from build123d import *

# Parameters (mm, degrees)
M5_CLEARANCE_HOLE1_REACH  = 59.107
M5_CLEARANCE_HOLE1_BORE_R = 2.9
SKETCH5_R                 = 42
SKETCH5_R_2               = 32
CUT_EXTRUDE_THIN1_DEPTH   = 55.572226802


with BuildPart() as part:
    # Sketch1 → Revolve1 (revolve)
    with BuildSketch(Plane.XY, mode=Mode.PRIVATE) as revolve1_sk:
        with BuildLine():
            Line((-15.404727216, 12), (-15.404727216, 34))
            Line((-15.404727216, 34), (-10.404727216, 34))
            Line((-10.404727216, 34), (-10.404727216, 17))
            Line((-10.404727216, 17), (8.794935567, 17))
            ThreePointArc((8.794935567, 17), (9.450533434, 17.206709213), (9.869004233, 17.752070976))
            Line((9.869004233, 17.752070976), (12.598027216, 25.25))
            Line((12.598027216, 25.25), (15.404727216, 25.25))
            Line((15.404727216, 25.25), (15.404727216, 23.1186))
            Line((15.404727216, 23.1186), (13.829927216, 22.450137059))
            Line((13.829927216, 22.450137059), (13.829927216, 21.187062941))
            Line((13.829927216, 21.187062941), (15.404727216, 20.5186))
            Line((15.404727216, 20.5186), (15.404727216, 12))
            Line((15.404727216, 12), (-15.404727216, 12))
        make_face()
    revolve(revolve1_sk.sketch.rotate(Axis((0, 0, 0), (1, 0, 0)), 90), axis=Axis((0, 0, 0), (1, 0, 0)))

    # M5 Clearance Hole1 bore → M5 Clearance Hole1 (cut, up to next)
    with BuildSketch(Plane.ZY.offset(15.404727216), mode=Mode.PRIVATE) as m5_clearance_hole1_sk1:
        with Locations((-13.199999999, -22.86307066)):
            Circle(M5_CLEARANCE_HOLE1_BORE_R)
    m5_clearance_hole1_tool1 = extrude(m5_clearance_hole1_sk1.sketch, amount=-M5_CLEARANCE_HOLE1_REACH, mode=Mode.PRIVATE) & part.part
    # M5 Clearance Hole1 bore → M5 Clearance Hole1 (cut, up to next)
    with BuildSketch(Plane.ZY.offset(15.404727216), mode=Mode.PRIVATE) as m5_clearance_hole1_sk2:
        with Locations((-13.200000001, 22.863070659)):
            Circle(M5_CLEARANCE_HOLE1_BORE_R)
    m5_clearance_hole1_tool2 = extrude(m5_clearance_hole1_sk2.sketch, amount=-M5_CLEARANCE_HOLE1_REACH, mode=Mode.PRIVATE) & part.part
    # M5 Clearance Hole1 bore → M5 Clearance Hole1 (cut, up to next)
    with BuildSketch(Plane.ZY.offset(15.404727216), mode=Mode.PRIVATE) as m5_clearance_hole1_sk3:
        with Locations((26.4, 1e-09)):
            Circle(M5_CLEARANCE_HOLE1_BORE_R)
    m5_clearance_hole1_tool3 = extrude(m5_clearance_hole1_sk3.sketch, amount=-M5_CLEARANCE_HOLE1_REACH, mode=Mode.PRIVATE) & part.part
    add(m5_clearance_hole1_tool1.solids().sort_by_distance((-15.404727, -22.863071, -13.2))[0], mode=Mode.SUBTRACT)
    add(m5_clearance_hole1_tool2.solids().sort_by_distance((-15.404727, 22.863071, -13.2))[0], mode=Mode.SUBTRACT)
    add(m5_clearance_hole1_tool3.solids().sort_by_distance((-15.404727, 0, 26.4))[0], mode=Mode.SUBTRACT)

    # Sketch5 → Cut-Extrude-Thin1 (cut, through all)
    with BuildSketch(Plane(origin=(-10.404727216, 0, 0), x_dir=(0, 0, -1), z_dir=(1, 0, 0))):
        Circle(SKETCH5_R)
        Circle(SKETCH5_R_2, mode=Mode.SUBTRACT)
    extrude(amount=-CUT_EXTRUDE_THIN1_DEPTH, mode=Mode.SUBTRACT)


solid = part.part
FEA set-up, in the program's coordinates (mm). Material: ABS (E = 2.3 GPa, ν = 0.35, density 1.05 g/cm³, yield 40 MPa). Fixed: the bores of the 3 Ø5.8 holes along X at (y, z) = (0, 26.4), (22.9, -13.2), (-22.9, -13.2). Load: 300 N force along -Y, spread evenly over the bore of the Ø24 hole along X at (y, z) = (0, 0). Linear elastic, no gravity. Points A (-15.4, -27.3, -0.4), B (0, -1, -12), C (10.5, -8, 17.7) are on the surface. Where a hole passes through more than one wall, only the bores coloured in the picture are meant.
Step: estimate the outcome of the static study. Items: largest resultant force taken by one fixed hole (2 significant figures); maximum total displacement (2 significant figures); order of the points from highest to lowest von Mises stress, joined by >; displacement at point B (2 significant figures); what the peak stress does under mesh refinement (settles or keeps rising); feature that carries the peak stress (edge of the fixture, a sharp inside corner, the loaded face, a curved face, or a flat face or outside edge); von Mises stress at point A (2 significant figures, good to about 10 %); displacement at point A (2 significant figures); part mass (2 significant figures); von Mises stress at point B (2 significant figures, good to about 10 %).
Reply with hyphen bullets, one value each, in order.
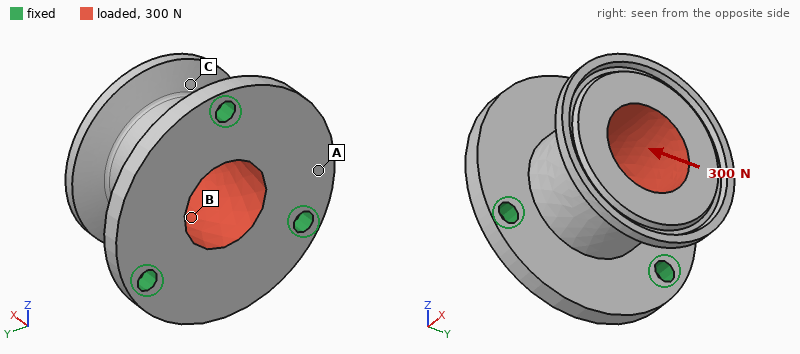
- 140 N
- 0.10 mm
- B > A > C
- 0.039 mm
- keeps rising
- edge of the fixture
- 1.0 MPa
- 0.028 mm
- 31 g
- 1.7 MPa
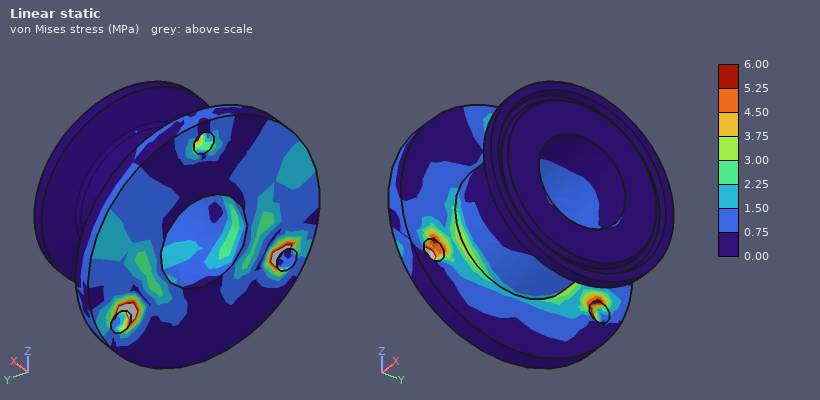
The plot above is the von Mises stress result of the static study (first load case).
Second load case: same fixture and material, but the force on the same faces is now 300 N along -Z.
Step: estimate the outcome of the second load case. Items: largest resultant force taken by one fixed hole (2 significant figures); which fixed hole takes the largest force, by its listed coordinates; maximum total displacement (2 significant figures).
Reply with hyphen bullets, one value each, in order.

- 150 N
- (0, 26.4)
- 0.11 mm
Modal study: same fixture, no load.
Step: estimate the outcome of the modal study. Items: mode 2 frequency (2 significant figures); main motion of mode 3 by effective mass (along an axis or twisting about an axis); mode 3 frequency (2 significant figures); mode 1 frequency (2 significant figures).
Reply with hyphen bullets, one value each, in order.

- 1800 Hz
- along X
- 2600 Hz
- 1800 Hz
